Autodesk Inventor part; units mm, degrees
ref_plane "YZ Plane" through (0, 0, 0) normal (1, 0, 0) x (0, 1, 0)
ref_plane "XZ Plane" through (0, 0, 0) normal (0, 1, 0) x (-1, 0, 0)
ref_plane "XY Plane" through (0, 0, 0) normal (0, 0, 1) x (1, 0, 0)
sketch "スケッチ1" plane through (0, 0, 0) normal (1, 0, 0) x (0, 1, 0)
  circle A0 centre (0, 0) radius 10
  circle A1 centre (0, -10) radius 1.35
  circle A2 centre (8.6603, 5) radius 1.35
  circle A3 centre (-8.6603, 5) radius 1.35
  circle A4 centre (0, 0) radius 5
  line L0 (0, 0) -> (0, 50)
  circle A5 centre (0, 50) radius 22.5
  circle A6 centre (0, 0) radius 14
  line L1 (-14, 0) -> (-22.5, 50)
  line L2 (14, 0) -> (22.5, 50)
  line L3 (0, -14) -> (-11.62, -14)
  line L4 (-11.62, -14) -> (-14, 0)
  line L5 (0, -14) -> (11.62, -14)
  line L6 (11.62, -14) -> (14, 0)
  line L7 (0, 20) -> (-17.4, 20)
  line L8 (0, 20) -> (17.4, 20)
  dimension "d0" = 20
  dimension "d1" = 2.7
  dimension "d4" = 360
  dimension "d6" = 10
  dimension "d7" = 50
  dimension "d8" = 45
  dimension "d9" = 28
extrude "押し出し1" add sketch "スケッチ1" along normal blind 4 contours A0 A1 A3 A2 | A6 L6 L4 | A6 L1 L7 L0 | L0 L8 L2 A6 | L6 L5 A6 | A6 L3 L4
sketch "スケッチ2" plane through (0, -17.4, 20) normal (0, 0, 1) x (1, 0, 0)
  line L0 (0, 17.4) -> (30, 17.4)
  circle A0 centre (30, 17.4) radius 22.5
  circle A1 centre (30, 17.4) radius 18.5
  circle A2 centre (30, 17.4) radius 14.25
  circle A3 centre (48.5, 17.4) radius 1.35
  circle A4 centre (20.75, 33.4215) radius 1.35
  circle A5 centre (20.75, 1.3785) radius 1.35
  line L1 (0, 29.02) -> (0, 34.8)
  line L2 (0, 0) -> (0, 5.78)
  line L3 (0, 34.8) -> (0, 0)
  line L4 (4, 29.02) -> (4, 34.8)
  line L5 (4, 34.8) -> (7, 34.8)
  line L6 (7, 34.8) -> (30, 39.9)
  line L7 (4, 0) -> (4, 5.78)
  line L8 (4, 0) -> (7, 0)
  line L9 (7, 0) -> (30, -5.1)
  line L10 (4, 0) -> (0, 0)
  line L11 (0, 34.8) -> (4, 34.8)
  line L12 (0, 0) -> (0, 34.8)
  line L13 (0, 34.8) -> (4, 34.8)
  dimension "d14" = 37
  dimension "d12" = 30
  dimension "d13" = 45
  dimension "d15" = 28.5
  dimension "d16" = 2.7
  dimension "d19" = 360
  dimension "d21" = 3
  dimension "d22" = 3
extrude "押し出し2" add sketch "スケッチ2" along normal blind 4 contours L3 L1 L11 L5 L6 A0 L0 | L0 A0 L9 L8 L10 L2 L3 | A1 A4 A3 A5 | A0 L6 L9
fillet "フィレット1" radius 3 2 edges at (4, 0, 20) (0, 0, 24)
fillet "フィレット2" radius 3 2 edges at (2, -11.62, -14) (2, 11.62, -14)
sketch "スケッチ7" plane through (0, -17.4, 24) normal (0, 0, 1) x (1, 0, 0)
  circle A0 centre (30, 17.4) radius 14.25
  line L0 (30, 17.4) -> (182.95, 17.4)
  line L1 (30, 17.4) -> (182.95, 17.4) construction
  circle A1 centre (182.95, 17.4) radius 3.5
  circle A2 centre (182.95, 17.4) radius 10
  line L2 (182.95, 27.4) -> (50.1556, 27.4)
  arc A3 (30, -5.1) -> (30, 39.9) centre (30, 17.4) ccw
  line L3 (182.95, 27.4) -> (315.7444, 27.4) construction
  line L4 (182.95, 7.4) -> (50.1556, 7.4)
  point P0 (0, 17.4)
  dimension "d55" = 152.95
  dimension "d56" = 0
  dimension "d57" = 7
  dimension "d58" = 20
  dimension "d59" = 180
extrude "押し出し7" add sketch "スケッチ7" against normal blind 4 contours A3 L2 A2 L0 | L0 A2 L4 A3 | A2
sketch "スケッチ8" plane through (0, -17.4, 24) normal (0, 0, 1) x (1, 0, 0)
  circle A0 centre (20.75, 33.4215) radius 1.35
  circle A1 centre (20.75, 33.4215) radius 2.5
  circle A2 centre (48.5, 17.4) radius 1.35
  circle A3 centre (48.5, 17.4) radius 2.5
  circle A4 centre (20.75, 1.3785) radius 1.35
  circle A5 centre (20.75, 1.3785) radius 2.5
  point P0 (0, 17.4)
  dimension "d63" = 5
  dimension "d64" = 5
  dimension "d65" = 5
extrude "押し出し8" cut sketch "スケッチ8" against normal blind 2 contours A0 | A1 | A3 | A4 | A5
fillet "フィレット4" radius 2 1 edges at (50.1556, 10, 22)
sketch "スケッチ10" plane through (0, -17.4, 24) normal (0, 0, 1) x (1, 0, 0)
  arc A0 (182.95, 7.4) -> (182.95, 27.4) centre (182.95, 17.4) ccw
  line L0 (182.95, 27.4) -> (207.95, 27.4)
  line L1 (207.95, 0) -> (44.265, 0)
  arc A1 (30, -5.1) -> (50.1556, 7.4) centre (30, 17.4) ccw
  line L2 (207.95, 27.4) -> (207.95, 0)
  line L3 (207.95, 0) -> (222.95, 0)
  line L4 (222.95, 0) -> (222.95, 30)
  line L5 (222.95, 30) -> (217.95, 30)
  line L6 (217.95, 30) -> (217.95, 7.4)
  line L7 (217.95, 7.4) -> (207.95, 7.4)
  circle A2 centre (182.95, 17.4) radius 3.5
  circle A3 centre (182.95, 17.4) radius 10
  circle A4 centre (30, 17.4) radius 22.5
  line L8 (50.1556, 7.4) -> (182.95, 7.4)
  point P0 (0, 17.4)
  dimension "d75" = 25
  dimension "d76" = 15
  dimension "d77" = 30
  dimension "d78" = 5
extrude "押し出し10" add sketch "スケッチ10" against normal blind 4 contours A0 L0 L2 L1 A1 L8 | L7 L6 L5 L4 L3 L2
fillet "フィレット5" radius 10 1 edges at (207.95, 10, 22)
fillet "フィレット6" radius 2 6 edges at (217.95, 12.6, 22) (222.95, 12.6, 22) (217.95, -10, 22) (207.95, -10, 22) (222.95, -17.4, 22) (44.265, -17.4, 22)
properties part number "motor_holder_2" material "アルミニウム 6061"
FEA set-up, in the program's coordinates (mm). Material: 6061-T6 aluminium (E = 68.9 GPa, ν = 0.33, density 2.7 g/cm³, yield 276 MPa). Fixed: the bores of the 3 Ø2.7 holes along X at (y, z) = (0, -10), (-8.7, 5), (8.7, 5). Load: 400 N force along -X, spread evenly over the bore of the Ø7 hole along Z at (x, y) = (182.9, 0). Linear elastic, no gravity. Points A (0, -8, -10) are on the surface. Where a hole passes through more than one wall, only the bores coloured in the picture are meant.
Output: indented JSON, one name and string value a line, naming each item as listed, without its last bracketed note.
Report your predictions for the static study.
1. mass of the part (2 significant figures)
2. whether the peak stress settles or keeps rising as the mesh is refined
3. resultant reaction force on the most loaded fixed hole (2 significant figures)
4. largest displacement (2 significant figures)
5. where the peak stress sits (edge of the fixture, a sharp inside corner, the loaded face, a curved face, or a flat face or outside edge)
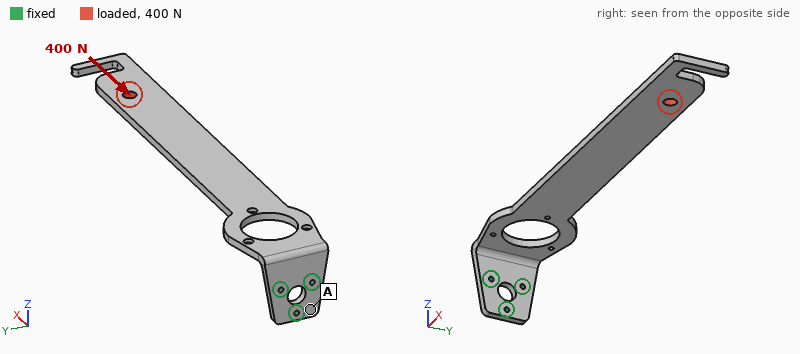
{
  "mass of the part": "72 g",
  "whether the peak stress settles or keeps rising as the mesh is refined": "keeps rising",
  "resultant reaction force on the most loaded fixed hole": "230 N",
  "largest displacement": "1.2 mm",
  "where the peak stress sits": "edge of the fixture"
}
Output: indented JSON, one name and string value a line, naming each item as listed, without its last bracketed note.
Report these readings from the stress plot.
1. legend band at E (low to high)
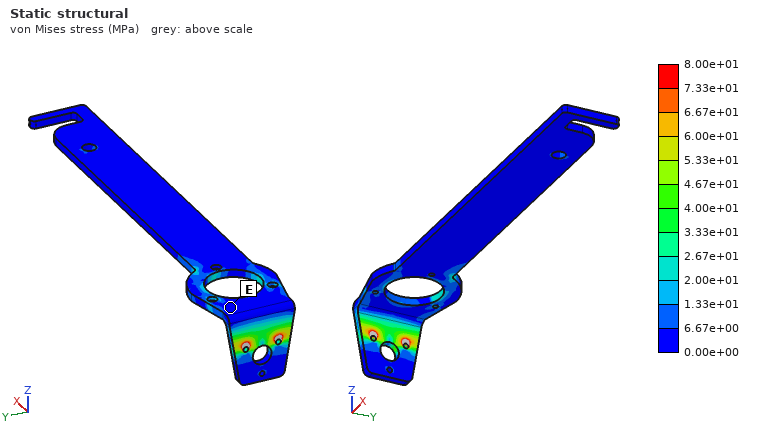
{
  "legend band at E": "0.00e+00 to 6.67e+00 MPa"
}
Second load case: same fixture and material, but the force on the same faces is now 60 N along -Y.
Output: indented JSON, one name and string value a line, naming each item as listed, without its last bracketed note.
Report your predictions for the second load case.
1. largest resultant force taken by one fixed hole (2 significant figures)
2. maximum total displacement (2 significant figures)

{
  "largest resultant force taken by one fixed hole": "520 N",
  "maximum total displacement": "1.3 mm"
}
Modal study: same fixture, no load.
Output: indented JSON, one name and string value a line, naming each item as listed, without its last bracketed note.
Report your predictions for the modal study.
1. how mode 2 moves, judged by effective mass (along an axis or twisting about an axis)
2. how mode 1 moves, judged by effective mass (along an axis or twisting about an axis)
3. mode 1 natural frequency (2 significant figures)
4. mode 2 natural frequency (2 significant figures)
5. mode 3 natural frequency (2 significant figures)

{
  "how mode 2 moves, judged by effective mass": "along Y",
  "how mode 1 moves, judged by effective mass": "along Z",
  "mode 1 natural frequency": "57 Hz",
  "mode 2 natural frequency": "230 Hz",
  "mode 3 natural frequency": "400 Hz"
}
